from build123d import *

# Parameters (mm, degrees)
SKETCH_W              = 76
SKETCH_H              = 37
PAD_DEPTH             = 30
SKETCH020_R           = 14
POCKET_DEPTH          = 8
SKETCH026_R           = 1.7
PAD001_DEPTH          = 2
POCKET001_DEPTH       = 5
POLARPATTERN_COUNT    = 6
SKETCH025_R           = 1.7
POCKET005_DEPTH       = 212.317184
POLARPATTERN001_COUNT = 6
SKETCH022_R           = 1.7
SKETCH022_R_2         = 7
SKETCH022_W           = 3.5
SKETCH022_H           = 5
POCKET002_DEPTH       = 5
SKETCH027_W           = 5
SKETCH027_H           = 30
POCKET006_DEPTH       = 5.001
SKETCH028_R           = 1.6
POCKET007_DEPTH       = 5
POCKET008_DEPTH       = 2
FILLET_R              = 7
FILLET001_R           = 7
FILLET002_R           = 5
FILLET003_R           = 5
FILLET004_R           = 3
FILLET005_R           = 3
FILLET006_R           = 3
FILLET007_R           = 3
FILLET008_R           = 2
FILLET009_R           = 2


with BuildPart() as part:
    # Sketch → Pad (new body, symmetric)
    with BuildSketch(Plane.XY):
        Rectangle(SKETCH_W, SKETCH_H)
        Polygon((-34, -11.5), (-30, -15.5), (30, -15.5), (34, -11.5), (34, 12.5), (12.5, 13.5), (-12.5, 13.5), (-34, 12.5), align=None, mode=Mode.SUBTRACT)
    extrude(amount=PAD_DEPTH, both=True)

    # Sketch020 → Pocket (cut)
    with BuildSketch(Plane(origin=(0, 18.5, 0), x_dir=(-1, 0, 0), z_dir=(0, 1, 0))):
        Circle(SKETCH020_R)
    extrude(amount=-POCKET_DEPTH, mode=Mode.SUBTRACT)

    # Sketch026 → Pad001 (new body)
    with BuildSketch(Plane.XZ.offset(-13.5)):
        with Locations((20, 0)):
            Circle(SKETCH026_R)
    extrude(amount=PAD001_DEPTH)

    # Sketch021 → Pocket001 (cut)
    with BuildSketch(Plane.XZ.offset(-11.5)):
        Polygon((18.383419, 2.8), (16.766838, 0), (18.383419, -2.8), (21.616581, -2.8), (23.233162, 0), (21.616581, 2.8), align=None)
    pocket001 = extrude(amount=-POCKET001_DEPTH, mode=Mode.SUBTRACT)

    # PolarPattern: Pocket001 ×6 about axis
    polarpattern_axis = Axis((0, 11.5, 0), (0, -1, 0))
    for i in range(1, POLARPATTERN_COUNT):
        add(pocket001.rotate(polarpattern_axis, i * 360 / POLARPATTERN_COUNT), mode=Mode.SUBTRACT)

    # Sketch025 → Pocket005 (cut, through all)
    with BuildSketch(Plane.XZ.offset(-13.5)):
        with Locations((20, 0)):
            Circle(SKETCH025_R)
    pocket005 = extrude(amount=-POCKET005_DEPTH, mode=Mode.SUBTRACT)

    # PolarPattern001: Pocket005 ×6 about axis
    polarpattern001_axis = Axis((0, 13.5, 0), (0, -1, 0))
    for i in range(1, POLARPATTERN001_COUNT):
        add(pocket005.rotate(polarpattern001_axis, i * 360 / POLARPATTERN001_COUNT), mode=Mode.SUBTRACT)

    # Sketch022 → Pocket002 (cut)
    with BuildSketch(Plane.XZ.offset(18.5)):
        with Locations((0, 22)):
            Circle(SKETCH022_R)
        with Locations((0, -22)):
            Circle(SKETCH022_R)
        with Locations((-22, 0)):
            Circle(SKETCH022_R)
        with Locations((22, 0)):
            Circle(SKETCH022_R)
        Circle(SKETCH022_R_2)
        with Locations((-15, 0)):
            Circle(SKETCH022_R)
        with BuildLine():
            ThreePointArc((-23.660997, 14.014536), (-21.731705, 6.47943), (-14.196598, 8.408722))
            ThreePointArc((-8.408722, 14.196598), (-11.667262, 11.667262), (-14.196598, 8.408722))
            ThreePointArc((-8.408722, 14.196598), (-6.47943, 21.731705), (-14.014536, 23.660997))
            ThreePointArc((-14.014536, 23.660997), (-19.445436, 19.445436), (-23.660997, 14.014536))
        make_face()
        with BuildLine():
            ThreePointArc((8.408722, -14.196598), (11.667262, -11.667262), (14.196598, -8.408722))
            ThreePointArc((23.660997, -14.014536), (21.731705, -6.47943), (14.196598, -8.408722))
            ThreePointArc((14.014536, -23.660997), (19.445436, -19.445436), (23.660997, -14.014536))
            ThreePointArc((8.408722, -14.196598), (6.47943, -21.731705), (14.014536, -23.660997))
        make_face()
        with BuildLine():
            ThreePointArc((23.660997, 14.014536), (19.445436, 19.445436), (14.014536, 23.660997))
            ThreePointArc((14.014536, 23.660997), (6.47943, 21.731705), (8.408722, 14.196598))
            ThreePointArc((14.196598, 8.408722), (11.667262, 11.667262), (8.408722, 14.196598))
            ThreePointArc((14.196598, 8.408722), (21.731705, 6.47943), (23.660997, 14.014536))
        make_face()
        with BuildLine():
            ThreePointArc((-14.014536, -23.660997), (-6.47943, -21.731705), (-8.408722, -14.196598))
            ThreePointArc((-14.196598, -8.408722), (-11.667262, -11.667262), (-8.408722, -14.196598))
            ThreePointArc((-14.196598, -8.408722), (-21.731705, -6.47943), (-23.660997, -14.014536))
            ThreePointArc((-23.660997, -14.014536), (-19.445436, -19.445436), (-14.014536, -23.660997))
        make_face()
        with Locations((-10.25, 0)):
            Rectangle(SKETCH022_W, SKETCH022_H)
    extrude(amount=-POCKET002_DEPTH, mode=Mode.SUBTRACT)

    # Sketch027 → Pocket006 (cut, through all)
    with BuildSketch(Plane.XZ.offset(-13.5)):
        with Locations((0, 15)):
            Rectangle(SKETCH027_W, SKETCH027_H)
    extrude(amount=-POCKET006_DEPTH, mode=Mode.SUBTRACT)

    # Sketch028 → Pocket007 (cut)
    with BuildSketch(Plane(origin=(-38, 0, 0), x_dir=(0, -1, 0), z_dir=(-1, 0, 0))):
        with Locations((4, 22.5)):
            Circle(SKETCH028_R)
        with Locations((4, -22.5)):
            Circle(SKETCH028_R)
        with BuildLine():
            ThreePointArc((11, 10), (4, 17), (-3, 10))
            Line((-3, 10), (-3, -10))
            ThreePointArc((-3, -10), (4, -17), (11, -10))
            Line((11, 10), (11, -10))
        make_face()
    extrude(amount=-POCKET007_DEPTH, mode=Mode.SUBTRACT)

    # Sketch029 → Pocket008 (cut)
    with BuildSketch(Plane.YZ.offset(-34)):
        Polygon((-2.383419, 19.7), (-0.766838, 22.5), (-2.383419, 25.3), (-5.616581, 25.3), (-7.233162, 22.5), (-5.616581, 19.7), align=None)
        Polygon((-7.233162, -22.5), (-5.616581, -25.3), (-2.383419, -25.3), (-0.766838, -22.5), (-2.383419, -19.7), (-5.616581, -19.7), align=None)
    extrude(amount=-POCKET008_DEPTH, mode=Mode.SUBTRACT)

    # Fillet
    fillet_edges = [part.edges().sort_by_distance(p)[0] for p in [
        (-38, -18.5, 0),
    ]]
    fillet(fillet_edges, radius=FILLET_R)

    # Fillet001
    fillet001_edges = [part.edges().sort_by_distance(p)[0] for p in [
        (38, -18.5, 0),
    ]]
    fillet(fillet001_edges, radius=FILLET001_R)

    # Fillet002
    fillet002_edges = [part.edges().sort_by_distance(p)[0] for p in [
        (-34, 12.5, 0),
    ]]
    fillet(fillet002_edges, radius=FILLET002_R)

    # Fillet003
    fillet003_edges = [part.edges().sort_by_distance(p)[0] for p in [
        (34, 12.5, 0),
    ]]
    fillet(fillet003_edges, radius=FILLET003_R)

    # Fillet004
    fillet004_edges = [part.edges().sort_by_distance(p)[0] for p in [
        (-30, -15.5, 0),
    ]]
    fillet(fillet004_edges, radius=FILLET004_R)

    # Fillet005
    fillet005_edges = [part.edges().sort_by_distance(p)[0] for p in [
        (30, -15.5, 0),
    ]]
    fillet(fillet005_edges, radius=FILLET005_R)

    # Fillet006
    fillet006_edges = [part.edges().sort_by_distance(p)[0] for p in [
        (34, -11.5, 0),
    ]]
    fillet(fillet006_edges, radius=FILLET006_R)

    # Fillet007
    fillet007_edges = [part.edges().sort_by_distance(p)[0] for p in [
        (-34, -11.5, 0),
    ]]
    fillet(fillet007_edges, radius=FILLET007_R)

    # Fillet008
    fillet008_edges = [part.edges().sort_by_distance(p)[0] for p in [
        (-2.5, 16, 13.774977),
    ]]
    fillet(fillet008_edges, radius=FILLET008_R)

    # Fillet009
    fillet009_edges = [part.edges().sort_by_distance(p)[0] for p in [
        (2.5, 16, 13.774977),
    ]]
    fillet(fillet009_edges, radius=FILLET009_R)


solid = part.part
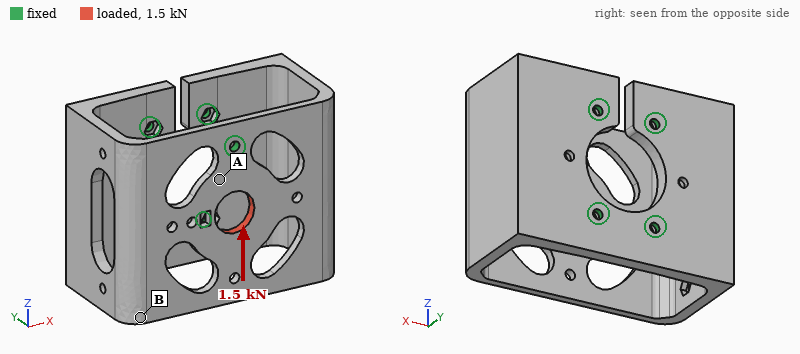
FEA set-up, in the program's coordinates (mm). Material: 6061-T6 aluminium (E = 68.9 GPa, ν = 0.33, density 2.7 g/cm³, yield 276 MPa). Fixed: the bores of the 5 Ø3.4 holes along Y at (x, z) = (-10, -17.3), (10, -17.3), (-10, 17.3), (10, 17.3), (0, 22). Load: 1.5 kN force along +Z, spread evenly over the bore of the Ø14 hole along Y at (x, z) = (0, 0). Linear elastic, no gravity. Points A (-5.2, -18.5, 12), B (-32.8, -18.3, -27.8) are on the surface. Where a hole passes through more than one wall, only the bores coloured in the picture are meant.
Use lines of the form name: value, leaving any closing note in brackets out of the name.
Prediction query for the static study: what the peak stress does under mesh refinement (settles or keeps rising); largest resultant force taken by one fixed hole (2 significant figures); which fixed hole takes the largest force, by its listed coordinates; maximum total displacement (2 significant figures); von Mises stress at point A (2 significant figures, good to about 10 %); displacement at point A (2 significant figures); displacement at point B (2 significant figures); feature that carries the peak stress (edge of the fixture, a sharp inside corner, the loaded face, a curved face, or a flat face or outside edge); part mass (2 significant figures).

what the peak stress does under mesh refinement: keeps rising
largest resultant force taken by one fixed hole: 1.4 kN
which fixed hole takes the largest force, by its listed coordinates: (0, 22)
maximum total displacement: 20 µm
von Mises stress at point A: 33 MPa
displacement at point A: 6.6 µm
displacement at point B: 13 µm
feature that carries the peak stress: edge of the fixture
part mass: 120 g
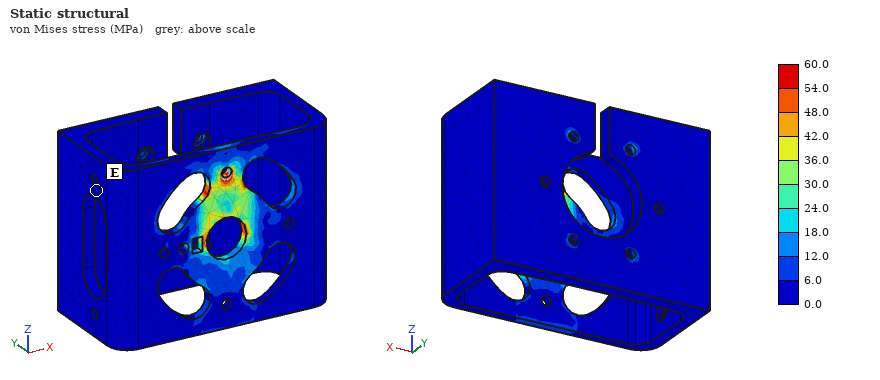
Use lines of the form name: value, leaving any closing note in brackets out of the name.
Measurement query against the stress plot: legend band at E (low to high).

legend band at E: 0.0 to 6.0 MPa
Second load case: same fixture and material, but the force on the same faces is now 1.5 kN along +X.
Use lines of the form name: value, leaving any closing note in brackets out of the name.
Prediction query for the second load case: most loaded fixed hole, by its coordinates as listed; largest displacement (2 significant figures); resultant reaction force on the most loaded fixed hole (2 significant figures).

most loaded fixed hole, by its coordinates as listed: (0, 22)
largest displacement: 90 µm
resultant reaction force on the most loaded fixed hole: 1.4 kN
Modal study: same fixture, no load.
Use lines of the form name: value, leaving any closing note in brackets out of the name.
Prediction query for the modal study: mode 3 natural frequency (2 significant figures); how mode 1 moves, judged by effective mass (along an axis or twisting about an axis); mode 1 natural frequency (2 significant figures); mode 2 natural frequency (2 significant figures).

mode 3 natural frequency: 3100 Hz
how mode 1 moves, judged by effective mass: along Y
mode 1 natural frequency: 2200 Hz
mode 2 natural frequency: 2300 Hz
